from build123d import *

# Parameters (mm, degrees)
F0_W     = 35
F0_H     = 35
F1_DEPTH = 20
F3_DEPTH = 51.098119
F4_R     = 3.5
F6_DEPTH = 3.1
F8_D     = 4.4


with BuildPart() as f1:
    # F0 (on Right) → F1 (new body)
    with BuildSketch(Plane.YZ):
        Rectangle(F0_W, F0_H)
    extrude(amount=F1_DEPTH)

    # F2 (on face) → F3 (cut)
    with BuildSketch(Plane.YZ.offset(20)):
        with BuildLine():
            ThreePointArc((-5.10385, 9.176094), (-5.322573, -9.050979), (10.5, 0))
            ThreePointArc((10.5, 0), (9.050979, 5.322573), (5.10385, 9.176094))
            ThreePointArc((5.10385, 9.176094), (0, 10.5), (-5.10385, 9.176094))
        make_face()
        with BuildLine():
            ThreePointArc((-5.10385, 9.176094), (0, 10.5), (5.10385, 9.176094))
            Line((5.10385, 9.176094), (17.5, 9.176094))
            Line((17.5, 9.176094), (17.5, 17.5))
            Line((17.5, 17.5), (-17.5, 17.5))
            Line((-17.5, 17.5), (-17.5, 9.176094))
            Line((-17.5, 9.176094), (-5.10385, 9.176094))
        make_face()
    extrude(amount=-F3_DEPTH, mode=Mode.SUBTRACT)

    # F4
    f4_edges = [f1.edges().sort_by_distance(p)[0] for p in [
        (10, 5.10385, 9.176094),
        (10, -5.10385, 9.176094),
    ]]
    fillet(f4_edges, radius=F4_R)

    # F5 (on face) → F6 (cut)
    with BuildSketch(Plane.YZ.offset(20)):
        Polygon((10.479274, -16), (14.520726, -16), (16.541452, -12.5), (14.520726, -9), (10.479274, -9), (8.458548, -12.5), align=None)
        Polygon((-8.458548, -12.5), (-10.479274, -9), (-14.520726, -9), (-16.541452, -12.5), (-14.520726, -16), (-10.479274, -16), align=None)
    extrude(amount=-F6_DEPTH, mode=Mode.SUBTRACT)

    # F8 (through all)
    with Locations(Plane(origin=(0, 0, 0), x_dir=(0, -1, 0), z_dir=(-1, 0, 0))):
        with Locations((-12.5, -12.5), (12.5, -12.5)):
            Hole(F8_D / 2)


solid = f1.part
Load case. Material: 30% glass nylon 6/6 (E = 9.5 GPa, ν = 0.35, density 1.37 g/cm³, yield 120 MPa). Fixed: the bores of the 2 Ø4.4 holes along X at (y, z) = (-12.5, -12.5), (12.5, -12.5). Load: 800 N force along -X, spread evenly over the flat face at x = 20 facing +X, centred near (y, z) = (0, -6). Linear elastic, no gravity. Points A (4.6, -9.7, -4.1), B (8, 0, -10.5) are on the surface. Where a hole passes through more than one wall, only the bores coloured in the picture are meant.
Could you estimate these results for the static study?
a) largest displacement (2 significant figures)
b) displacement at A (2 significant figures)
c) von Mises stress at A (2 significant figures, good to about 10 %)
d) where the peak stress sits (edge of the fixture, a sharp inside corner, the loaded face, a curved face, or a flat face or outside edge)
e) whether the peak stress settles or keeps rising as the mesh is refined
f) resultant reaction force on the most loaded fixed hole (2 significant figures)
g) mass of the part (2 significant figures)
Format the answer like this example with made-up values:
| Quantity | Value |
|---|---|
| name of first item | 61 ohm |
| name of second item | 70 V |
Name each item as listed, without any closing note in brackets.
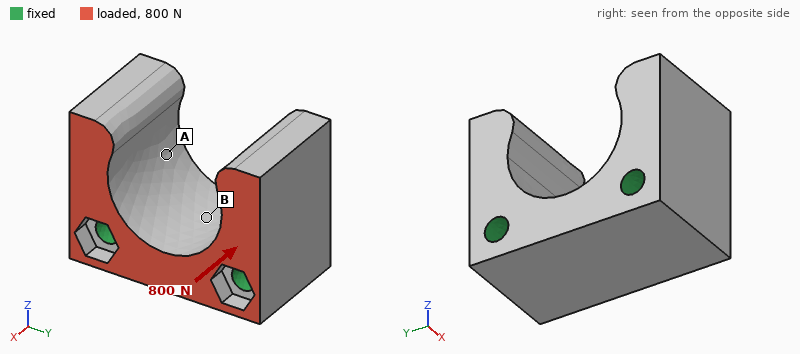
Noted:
| Quantity | Value |
|---|---|
| largest displacement | 17 µm |
| displacement at A | 4.1 µm |
| von Mises stress at A | 3.5 MPa |
| where the peak stress sits | edge of the fixture |
| whether the peak stress settles or keeps rising as the mesh is refined | keeps rising |
| resultant reaction force on the most loaded fixed hole | 400 N |
| mass of the part | 15 g |
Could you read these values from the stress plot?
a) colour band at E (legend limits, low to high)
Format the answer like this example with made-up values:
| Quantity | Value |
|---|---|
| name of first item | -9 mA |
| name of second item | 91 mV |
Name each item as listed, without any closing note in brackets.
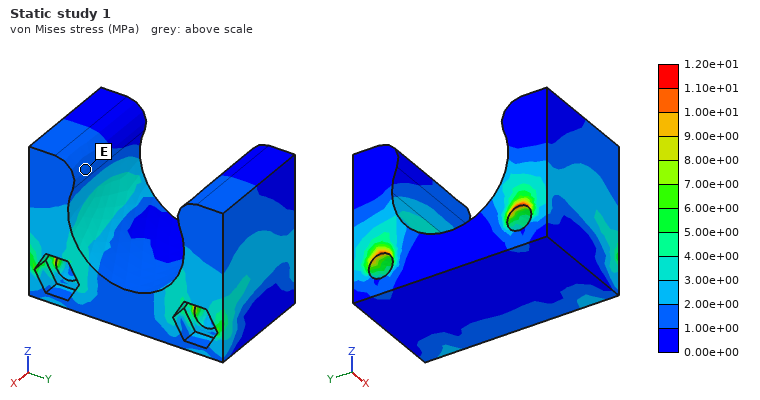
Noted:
| Quantity | Value |
|---|---|
| colour band at E | 1.00e+00 to 2.00e+00 MPa |
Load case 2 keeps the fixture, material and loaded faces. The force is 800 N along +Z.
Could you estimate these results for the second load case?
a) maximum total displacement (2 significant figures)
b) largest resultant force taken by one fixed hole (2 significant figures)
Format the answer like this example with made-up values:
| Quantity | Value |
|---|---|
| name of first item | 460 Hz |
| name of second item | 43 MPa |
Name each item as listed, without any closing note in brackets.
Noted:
| Quantity | Value |
|---|---|
| maximum total displacement | 22 µm |
| largest resultant force taken by one fixed hole | 400 N |
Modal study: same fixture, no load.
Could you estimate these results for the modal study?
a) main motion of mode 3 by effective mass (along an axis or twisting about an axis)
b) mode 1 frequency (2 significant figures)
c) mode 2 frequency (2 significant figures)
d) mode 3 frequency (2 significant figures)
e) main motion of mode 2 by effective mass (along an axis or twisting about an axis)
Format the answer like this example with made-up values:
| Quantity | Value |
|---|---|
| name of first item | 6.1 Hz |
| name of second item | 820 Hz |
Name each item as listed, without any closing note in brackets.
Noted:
| Quantity | Value |
|---|---|
| main motion of mode 3 by effective mass | along X |
| mode 1 frequency | 7500 Hz |
| mode 2 frequency | 8100 Hz |
| mode 3 frequency | 12 kHz |
| main motion of mode 2 by effective mass | along Y |
